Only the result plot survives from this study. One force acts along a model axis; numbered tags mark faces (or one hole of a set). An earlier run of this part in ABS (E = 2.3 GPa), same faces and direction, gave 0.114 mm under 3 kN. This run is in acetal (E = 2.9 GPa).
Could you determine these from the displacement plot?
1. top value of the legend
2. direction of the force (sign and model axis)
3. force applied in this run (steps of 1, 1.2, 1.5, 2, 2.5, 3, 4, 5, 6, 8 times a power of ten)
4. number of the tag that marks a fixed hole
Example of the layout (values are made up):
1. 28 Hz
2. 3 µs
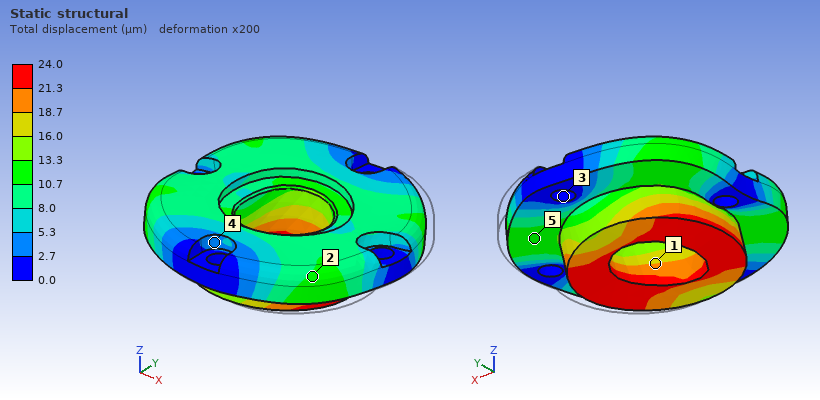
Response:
1. 24.0 µm
2. -X
3. 800 N
4. 3
